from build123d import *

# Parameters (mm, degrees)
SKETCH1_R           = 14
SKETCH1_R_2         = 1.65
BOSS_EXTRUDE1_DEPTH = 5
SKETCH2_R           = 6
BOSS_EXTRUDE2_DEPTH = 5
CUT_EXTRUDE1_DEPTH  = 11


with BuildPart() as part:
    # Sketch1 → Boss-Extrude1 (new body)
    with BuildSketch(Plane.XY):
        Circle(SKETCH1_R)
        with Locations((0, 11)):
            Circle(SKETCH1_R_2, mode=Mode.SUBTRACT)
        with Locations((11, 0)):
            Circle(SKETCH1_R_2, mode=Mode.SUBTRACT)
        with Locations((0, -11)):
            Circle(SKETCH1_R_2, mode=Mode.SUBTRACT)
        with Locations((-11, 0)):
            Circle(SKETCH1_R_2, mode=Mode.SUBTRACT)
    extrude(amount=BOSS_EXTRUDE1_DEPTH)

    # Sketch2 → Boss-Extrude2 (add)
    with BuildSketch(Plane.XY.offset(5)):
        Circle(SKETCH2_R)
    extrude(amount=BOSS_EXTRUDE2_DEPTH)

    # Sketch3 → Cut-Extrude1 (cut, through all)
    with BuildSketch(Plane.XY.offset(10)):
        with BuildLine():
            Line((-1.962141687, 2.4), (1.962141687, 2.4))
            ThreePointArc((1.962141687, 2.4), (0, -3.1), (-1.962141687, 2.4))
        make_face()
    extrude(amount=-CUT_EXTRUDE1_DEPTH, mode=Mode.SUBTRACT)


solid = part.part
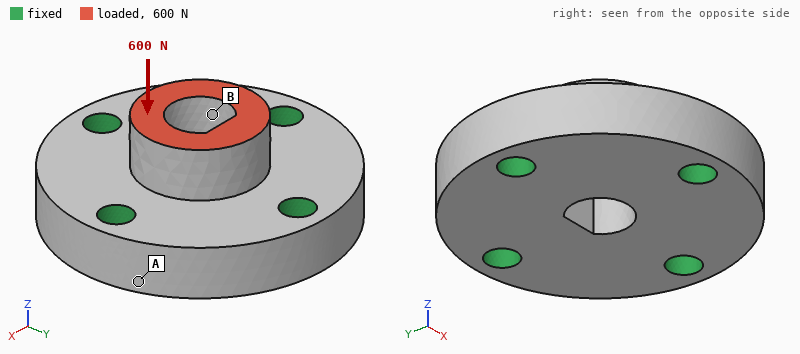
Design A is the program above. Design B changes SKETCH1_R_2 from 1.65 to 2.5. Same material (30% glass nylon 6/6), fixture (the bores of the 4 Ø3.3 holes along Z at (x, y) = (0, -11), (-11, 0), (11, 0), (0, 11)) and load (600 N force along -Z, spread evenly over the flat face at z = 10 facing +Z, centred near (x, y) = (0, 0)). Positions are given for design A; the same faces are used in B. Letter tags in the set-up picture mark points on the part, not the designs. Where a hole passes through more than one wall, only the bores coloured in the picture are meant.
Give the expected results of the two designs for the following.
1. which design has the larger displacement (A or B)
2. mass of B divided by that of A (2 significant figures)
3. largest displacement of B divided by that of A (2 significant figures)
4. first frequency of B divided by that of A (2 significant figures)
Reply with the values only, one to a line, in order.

A
0.93
0.81
1.2
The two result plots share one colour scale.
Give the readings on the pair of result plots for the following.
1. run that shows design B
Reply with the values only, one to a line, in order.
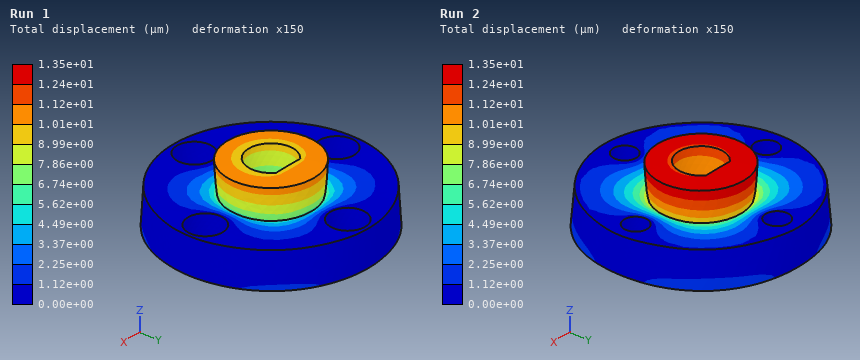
Run 1
